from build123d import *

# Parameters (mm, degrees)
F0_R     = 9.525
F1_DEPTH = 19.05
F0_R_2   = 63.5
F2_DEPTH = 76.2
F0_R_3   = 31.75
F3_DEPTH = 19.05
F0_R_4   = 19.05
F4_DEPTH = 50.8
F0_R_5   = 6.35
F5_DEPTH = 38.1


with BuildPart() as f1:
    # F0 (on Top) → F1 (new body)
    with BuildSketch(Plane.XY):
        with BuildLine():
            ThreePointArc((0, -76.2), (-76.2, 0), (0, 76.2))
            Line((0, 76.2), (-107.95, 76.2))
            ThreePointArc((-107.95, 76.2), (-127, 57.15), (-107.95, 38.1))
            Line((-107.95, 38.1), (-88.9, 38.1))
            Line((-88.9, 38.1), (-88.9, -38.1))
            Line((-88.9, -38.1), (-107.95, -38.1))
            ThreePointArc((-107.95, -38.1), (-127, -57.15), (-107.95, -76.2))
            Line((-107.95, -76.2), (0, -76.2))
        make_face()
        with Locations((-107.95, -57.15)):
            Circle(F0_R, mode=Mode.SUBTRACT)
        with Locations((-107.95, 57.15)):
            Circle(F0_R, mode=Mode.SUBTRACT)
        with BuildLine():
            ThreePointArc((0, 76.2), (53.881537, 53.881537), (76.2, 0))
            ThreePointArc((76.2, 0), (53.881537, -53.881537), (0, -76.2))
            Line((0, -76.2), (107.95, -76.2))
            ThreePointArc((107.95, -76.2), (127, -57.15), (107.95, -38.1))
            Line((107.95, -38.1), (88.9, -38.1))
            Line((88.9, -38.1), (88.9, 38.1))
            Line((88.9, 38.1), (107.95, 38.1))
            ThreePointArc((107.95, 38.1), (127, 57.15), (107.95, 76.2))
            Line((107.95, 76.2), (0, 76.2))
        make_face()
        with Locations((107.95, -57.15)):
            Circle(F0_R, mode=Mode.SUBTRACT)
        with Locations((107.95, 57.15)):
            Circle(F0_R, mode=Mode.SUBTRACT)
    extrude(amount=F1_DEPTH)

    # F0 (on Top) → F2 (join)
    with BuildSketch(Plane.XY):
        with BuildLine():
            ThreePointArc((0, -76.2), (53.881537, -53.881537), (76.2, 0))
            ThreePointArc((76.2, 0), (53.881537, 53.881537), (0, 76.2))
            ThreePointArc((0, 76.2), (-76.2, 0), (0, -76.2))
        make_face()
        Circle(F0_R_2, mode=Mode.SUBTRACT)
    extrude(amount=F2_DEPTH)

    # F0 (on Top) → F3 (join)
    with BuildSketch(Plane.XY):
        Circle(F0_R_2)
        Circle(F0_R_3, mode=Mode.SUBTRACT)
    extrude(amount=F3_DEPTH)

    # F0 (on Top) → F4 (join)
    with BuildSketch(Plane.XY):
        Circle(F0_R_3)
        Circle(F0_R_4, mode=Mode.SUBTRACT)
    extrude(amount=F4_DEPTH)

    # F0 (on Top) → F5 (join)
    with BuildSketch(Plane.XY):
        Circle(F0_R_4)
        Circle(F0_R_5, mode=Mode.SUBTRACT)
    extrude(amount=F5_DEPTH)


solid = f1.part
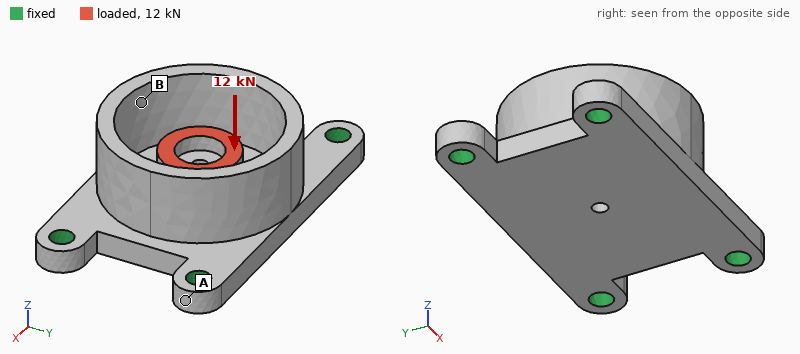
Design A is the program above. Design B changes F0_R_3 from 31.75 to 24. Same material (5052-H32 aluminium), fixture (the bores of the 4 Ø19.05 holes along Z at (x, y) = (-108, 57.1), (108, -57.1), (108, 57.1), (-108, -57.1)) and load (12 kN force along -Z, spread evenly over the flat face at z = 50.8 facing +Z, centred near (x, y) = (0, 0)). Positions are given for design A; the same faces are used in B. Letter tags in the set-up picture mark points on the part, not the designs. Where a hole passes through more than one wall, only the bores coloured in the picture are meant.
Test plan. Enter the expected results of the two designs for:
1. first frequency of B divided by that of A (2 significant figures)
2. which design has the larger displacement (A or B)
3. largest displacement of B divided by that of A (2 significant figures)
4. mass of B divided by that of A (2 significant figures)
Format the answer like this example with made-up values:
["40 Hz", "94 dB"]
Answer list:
["1.0", "B", "1.2", "0.96"]
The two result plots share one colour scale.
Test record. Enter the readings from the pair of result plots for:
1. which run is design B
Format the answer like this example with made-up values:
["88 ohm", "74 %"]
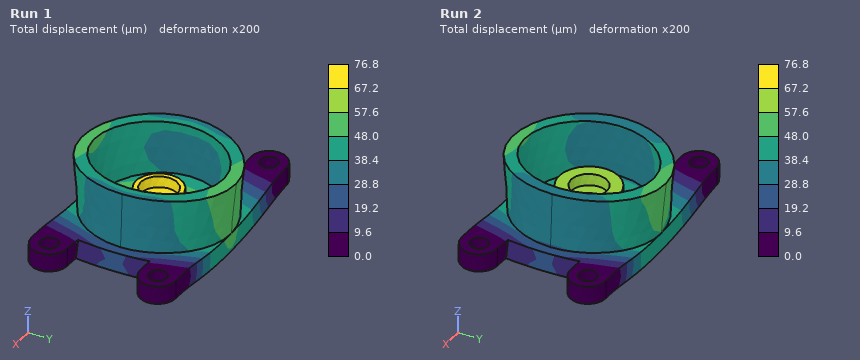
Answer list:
["Run 1"]
